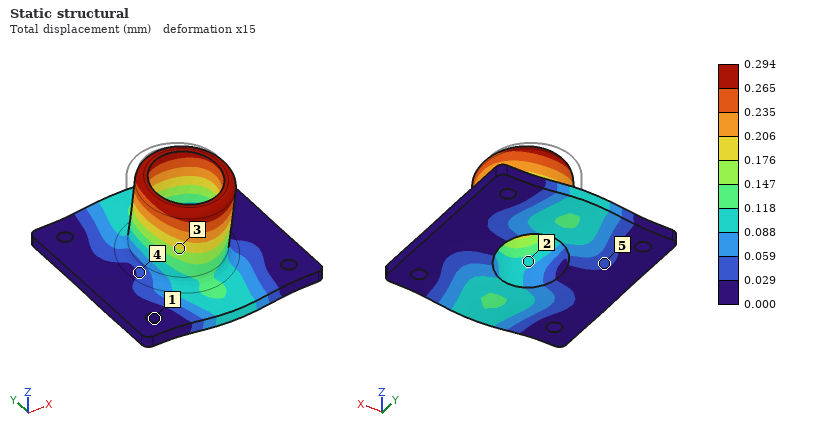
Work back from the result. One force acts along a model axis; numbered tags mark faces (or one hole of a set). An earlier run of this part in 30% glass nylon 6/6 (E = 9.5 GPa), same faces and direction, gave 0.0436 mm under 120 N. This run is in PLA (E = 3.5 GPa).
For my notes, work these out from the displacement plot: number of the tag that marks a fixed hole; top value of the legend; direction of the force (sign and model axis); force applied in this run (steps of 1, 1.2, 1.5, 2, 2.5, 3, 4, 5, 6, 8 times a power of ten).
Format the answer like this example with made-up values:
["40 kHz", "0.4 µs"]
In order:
["1", "0.294 mm", "-Y", "300 N"]
